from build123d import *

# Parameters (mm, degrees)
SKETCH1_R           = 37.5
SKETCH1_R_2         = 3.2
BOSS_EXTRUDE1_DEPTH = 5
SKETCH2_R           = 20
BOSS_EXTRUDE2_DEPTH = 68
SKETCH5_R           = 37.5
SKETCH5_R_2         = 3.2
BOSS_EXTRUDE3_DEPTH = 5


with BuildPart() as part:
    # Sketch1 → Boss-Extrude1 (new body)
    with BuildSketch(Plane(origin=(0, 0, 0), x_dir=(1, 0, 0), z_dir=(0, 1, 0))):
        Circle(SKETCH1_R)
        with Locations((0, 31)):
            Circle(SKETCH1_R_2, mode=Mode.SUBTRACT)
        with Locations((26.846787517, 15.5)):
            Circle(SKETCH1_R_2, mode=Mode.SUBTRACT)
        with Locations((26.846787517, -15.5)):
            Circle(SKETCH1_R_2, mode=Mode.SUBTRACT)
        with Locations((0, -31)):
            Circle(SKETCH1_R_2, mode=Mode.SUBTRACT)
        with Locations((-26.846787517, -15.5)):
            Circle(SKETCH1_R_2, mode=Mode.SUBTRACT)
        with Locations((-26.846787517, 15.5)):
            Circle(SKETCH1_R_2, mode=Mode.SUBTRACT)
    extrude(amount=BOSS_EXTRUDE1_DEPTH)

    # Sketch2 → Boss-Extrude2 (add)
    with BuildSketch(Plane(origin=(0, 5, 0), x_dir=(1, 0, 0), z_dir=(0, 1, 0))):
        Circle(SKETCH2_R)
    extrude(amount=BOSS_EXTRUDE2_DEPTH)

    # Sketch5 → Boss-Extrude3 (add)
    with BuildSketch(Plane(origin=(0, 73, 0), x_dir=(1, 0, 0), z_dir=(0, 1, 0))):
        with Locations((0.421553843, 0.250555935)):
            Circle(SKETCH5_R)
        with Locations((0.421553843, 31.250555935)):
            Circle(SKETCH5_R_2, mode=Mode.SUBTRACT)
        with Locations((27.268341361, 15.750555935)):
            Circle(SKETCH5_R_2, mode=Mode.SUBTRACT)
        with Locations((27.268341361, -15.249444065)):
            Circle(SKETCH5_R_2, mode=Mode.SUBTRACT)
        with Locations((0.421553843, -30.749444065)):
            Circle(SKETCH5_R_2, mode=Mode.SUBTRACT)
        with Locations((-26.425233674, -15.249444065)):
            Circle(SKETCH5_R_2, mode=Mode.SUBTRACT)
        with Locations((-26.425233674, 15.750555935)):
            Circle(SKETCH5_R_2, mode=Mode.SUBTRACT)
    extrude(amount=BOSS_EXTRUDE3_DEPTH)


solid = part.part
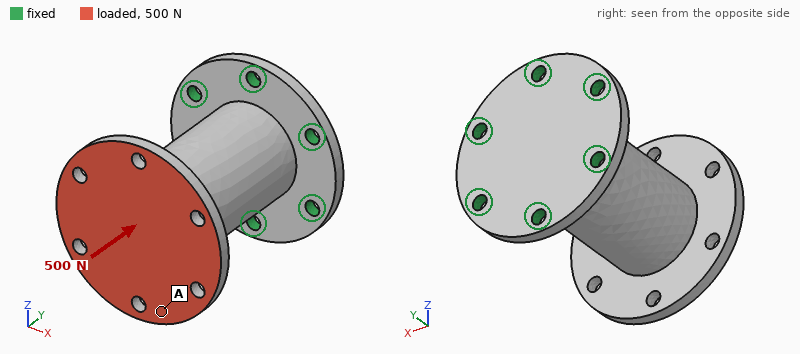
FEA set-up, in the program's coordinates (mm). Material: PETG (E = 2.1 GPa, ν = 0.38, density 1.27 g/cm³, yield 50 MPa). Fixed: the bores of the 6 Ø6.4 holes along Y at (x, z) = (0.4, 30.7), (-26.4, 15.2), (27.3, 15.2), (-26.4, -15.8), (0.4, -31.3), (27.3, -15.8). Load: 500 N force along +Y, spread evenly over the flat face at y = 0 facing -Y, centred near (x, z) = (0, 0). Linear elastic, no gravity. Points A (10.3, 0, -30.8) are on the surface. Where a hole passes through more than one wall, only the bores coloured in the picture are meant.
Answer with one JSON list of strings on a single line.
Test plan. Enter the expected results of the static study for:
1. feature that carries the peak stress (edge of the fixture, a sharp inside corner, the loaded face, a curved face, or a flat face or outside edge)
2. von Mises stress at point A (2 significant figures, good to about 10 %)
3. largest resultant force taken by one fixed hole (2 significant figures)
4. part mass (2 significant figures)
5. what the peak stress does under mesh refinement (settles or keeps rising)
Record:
["edge of the fixture", "0.96 MPa", "93 N", "160 g", "keeps rising"]
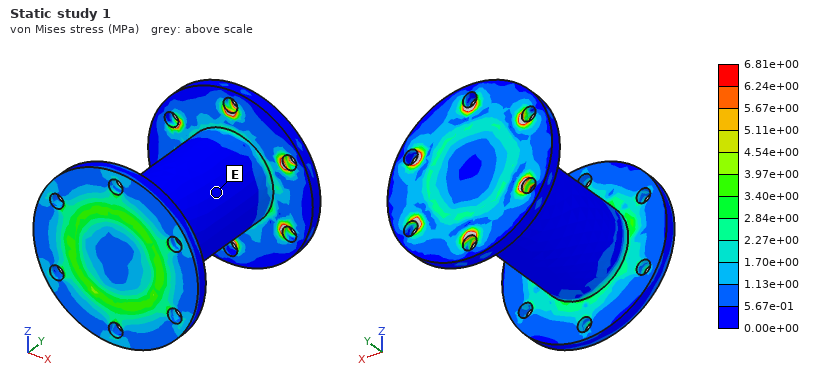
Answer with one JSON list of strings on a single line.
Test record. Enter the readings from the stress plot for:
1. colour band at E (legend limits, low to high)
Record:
["0.00e+00 to 5.67e-01 MPa"]
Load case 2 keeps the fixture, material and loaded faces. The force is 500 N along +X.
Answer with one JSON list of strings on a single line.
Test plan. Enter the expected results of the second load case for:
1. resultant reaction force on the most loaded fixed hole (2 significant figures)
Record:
["460 N"]
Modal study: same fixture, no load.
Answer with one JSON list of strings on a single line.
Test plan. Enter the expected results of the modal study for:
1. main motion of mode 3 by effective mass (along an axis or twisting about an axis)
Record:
["along Y"]
